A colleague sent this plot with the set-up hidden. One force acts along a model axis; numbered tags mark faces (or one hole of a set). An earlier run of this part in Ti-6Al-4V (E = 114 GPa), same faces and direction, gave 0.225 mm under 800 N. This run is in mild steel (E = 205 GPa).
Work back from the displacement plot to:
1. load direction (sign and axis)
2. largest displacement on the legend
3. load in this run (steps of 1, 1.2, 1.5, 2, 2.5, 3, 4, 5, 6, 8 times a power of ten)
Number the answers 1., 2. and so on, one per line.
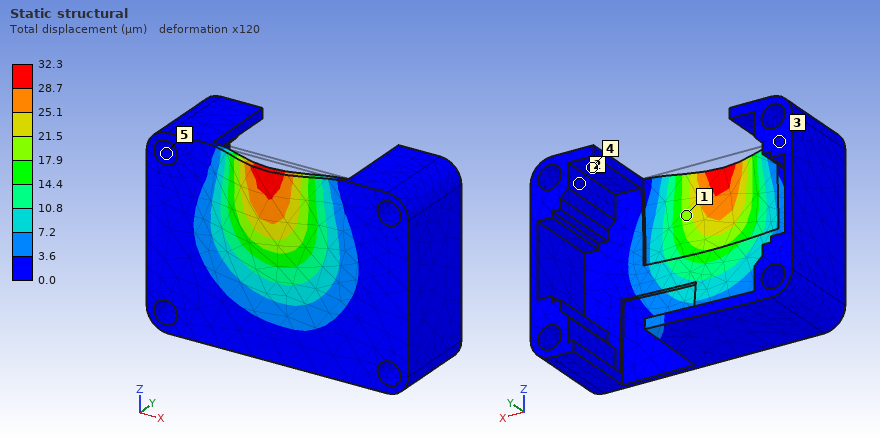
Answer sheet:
1. -Y
2. 32.3 µm
3. 200 N
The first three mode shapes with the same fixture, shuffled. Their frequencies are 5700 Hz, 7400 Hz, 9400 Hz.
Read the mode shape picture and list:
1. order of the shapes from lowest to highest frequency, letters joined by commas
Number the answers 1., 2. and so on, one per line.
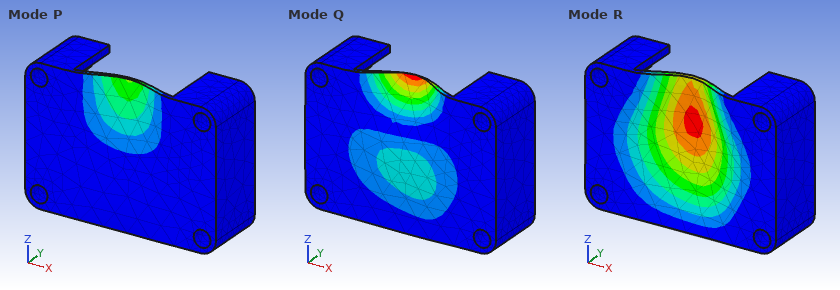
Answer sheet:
1. R, P, Q
